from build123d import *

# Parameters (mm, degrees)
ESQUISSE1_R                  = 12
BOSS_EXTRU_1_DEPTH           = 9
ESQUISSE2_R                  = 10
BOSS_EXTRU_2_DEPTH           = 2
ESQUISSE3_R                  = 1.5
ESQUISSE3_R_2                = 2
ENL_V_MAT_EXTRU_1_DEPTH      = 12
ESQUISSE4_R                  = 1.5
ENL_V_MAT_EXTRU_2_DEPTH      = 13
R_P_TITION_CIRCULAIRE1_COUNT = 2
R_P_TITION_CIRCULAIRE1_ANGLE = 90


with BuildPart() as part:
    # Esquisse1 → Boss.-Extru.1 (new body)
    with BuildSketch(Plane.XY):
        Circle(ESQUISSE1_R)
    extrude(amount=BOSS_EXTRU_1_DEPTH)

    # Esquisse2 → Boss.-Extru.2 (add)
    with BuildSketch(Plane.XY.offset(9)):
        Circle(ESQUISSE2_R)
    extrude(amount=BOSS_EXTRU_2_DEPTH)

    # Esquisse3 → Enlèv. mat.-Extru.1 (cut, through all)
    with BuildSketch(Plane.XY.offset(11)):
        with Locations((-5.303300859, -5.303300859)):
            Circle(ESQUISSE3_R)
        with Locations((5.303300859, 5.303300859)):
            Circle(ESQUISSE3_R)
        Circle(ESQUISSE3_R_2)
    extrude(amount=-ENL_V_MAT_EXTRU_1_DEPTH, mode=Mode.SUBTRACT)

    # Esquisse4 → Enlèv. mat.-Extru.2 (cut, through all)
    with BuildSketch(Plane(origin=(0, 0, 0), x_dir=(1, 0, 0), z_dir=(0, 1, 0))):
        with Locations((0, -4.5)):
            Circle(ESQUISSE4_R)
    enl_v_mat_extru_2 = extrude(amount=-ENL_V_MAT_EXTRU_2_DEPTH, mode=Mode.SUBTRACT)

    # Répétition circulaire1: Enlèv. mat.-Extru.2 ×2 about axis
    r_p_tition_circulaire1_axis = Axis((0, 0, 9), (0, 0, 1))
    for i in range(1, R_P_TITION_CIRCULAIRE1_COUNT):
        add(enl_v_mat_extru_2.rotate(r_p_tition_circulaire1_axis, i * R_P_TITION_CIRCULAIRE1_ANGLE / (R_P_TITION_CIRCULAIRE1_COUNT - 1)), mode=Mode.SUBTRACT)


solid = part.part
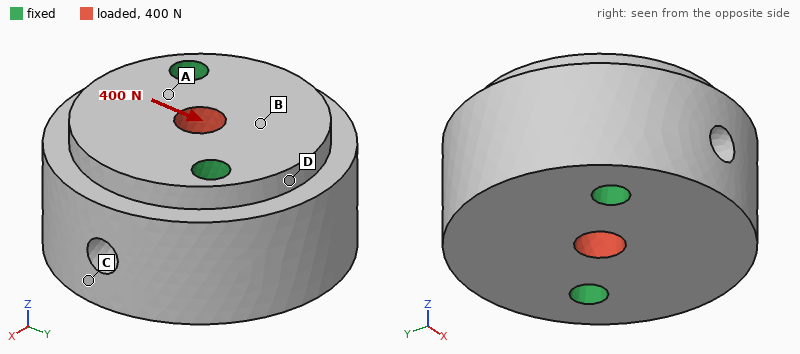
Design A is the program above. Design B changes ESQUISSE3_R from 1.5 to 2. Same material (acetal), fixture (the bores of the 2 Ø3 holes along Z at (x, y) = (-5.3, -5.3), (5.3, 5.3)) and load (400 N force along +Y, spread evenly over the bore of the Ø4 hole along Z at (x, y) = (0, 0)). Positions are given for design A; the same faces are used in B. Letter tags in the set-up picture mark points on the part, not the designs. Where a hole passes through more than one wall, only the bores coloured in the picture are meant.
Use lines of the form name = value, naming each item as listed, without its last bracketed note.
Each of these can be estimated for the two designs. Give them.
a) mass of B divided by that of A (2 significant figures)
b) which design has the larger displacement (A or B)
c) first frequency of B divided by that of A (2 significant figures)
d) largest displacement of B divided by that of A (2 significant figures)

mass of B divided by that of A = 0.97
which design has the larger displacement = A
first frequency of B divided by that of A = 1.1
largest displacement of B divided by that of A = 0.90
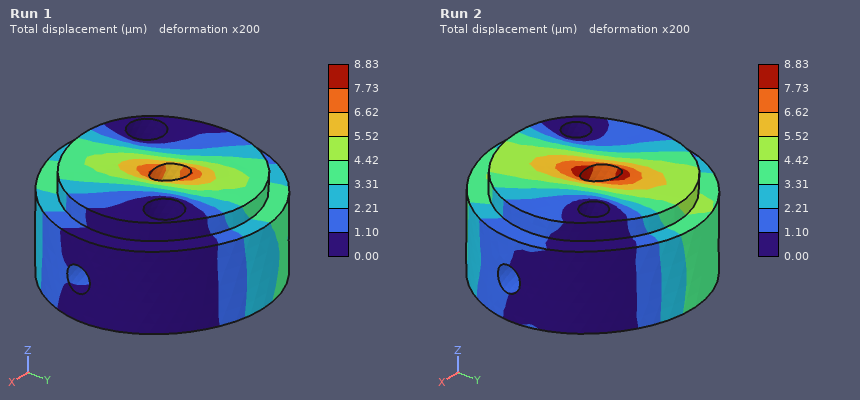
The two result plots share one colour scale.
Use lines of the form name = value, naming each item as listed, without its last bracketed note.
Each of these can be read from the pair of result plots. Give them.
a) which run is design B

which run is design B = Run 1
